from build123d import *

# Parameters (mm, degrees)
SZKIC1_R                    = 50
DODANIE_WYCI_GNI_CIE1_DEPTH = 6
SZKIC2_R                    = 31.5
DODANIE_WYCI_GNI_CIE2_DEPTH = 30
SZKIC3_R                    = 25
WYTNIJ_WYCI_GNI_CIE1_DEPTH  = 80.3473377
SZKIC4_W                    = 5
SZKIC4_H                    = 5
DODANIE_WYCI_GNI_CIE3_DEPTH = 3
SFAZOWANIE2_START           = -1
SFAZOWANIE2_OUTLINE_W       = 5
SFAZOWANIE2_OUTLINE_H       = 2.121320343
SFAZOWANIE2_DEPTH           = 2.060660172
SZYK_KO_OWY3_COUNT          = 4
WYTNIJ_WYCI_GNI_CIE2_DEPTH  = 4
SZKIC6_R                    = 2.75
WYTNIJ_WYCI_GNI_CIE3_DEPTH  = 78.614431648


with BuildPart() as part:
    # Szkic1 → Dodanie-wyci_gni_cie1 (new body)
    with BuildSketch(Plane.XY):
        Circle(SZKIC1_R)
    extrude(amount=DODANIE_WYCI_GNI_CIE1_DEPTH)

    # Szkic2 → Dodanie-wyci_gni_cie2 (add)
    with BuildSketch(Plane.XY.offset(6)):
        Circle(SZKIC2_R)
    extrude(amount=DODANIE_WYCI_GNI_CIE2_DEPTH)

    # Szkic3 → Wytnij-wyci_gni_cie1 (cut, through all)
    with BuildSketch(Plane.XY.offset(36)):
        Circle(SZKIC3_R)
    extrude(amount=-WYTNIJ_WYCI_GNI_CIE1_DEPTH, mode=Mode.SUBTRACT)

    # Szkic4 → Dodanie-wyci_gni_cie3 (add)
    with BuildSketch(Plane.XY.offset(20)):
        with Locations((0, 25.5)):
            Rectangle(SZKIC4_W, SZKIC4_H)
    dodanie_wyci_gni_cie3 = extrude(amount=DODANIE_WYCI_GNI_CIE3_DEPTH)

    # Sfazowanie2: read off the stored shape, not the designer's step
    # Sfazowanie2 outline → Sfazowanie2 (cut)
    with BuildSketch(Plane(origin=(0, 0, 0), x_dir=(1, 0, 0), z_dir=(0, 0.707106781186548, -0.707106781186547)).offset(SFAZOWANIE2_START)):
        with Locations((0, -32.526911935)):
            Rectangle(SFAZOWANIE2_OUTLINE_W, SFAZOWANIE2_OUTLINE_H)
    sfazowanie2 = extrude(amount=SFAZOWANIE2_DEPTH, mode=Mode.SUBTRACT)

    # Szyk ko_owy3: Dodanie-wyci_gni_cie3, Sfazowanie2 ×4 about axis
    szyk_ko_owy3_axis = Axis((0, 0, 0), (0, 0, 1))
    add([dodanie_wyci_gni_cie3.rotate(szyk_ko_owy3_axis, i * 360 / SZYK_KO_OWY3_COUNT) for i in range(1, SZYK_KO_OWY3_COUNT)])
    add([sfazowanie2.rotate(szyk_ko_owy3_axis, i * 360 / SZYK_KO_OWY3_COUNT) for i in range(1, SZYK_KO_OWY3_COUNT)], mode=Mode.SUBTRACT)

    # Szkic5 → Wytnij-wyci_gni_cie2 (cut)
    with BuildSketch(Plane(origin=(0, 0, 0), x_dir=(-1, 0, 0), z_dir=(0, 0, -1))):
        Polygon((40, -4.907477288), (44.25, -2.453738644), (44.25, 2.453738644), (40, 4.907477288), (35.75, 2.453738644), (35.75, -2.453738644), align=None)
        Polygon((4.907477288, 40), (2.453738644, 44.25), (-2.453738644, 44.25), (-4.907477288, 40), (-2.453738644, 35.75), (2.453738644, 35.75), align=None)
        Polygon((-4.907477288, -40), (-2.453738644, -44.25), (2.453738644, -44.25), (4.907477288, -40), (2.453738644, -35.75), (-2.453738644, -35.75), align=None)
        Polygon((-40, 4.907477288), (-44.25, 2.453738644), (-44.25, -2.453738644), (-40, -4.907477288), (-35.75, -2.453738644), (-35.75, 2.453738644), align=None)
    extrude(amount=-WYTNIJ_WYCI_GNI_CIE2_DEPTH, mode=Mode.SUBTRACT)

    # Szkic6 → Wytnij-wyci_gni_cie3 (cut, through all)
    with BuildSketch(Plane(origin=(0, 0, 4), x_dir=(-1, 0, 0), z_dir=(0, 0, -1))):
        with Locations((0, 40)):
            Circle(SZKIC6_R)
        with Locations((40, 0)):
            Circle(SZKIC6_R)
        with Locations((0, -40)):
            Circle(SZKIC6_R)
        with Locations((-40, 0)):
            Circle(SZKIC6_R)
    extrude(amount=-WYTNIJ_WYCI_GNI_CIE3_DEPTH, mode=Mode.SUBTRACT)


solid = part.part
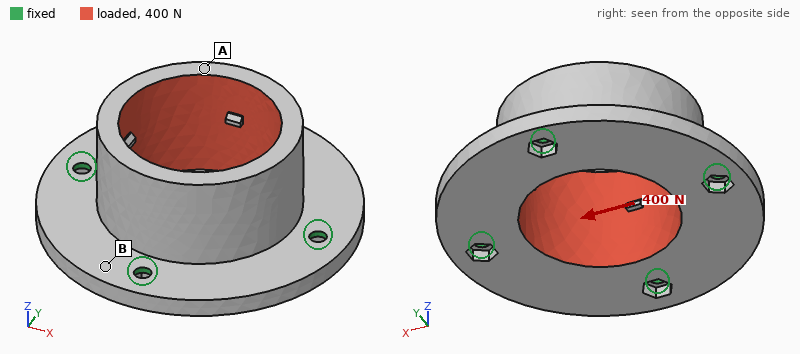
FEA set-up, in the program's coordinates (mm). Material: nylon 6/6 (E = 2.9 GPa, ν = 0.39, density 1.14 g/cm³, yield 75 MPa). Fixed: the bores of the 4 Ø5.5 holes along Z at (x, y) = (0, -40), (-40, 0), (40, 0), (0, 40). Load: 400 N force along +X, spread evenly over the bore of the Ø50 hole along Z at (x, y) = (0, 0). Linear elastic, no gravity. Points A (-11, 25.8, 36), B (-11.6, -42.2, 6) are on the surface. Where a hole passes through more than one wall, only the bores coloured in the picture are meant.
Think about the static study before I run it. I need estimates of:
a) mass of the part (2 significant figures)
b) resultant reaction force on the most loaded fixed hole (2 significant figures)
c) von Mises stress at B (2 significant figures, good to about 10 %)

78 g
120 N
0.83 MPa
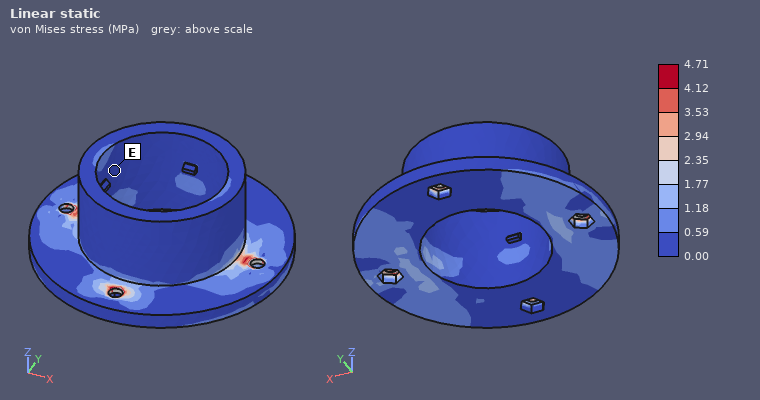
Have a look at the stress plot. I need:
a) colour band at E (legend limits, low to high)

0.00 to 0.59 MPa
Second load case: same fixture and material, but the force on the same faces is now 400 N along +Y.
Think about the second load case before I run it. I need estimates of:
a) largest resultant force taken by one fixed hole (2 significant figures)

120 N
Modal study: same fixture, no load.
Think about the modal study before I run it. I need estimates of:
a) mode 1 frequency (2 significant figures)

1700 Hz
